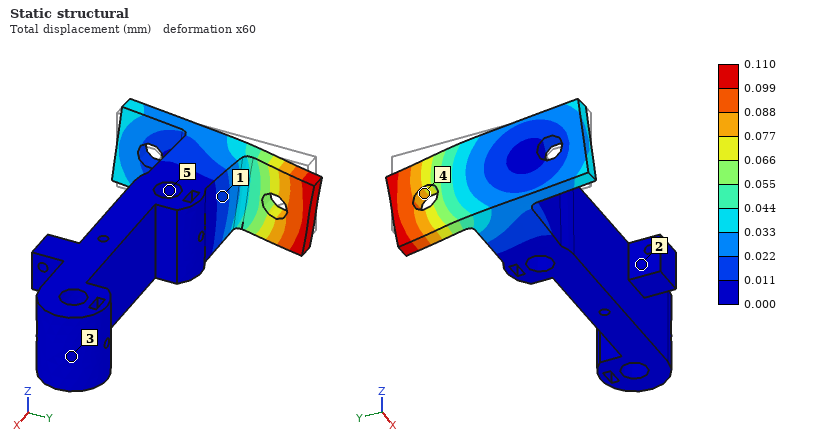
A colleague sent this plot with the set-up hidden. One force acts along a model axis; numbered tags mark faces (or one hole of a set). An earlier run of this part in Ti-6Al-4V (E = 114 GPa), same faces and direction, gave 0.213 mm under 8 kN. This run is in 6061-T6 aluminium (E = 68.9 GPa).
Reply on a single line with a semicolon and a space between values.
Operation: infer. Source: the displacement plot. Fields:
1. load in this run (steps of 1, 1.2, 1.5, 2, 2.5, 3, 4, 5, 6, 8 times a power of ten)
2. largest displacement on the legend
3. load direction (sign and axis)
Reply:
2.5 kN; 0.110 mm; -Z
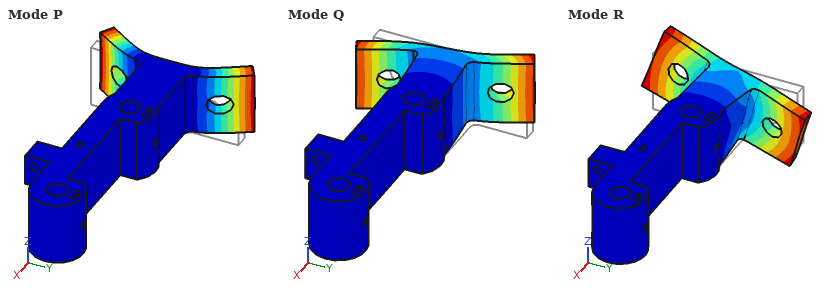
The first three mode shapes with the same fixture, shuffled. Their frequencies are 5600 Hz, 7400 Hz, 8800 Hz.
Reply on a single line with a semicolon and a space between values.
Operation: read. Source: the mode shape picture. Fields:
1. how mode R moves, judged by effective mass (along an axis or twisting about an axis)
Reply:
twisting about X
